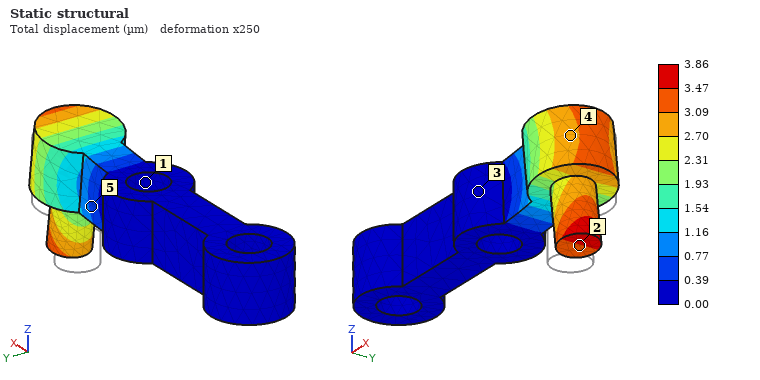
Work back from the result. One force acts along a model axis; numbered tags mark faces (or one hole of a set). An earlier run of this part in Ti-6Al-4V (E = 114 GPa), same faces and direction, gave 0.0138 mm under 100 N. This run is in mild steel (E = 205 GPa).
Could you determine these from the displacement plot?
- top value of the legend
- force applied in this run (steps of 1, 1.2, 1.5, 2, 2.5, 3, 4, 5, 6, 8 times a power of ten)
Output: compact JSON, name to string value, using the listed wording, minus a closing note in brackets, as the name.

{"top value of the legend": "3.86 µm", "force applied in this run": "50 N"}
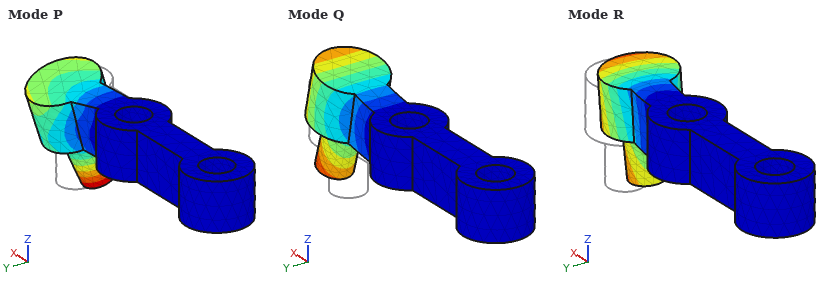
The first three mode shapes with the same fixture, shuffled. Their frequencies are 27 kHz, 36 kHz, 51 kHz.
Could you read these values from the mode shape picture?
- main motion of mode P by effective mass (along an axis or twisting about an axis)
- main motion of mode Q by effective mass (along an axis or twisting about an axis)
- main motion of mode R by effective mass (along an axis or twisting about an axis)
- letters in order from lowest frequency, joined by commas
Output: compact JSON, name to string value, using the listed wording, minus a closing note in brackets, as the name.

{"main motion of mode P by effective mass": "twisting about X", "main motion of mode Q by effective mass": "along Z", "main motion of mode R by effective mass": "along Y", "letters in order from lowest frequency, joined by commas": "R, Q, P"}
